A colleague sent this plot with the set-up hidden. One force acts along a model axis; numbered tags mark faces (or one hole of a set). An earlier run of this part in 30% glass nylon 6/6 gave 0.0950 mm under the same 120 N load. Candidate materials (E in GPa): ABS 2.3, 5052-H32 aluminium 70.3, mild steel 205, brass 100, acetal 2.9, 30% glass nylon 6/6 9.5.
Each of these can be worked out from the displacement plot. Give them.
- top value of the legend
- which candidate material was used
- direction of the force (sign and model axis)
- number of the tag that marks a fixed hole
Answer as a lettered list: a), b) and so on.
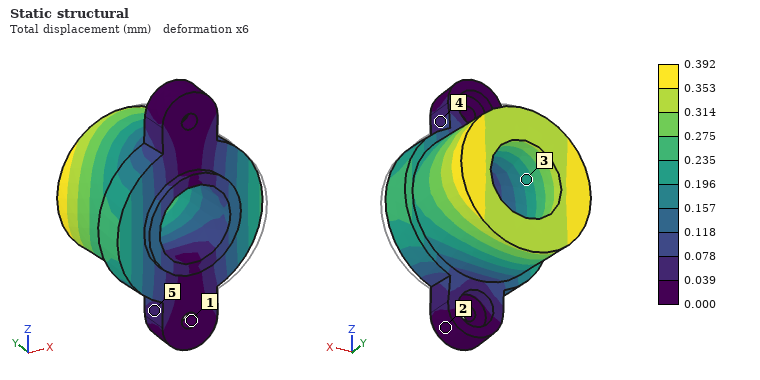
a) 0.392 mm
b) ABS
c) -X
d) 1
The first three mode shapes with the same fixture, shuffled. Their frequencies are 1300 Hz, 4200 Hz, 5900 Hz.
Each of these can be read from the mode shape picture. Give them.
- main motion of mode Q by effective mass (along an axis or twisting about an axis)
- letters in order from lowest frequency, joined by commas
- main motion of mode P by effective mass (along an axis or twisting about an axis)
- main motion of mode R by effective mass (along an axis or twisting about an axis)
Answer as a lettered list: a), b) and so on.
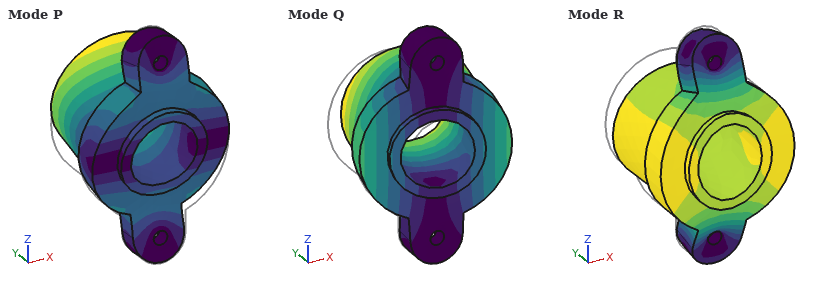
a) along X
b) Q, R, P
c) along Z
d) along Y
